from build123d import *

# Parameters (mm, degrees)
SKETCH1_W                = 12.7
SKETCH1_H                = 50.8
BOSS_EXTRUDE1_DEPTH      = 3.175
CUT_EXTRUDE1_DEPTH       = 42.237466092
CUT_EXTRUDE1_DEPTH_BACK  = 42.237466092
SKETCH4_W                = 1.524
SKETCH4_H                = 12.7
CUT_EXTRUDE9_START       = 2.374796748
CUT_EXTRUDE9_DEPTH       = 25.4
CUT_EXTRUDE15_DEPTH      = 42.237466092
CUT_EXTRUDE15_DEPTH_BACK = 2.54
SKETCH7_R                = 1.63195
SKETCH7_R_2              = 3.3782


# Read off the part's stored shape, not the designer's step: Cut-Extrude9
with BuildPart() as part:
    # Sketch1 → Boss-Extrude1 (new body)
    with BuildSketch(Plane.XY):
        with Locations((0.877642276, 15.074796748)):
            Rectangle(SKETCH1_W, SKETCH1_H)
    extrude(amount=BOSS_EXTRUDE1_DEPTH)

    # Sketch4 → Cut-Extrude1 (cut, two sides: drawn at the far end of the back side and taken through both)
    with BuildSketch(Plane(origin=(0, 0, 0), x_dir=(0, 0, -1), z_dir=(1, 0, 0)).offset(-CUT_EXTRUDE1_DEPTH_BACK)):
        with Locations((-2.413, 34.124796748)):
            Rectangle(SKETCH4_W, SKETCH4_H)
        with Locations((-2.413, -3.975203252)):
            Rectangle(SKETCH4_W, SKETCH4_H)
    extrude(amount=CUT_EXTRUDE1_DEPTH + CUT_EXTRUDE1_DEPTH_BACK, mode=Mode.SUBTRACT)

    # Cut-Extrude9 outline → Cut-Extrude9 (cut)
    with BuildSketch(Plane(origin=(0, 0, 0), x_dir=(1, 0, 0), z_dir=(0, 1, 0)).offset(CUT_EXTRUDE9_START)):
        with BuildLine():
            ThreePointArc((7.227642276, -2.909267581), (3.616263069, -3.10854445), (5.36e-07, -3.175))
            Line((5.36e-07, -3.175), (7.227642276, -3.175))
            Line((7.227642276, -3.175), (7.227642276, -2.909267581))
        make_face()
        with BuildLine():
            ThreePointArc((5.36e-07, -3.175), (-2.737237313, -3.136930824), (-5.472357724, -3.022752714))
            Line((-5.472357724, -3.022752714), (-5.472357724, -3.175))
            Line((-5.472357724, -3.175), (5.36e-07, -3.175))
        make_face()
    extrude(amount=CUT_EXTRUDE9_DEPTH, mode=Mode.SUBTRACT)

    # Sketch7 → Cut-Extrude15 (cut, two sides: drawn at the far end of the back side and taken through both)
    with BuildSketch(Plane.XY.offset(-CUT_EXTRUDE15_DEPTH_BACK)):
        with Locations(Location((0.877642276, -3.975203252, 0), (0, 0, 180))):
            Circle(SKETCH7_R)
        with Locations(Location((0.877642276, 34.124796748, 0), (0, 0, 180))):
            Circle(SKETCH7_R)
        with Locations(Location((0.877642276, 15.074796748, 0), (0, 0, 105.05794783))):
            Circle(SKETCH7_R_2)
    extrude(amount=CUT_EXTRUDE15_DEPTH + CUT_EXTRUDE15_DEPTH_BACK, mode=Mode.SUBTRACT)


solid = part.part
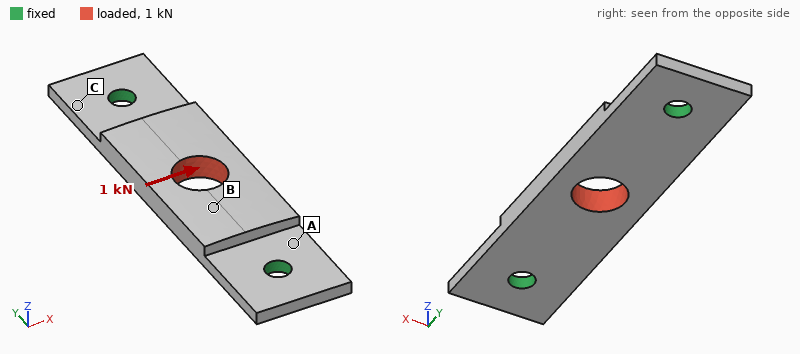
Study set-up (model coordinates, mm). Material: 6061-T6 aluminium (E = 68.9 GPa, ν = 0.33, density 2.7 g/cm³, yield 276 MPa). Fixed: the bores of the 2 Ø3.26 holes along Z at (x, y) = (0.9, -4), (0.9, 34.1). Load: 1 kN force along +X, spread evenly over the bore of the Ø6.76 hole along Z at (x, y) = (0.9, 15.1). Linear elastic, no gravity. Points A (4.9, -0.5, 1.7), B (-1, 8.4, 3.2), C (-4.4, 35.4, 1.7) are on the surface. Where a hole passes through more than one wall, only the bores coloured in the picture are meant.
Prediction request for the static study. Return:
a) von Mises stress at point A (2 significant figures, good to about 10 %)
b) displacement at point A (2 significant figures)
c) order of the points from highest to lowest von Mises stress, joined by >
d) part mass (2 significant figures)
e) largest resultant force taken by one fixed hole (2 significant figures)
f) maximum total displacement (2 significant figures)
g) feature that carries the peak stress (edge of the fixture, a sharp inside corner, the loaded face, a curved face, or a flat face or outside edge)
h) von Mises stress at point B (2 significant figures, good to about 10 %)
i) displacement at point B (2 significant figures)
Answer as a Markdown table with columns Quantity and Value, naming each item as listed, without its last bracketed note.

| Quantity | Value |
|---|---|
| von Mises stress at point A | 59 MPa |
| displacement at point A | 13 µm |
| order of the points from highest to lowest von Mises stress, joined by > | A > B > C |
| part mass | 3.8 g |
| largest resultant force taken by one fixed hole | 500 N |
| maximum total displacement | 47 µm |
| feature that carries the peak stress | edge of the fixture |
| von Mises stress at point B | 34 MPa |
| displacement at point B | 36 µm |
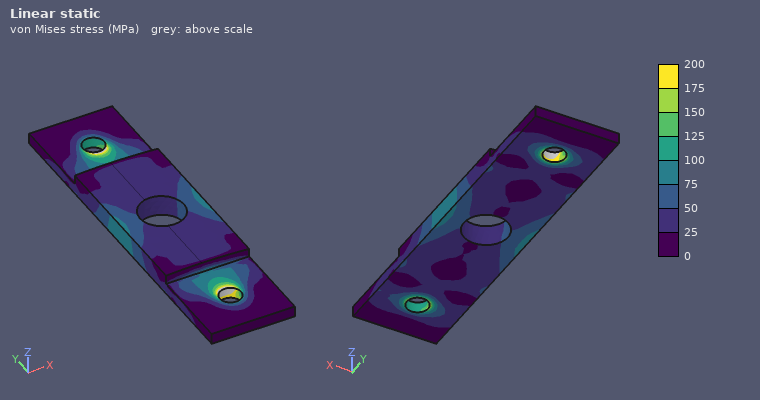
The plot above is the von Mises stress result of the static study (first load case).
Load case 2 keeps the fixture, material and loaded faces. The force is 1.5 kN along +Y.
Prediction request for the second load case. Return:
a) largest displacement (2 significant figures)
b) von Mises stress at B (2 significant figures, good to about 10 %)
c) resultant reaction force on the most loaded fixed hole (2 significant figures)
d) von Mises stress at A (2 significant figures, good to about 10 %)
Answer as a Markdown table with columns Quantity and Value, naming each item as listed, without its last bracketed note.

| Quantity | Value |
|---|---|
| largest displacement | 9.1 µm |
| von Mises stress at B | 13 MPa |
| resultant reaction force on the most loaded fixed hole | 750 N |
| von Mises stress at A | 36 MPa |
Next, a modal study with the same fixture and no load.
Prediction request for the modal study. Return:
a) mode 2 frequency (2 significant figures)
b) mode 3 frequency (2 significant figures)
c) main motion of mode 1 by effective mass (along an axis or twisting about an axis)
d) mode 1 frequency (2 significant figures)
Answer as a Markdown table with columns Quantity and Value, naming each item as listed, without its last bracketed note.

| Quantity | Value |
|---|---|
| mode 2 frequency | 11 kHz |
| mode 3 frequency | 20 kHz |
| main motion of mode 1 by effective mass | along Z |
| mode 1 frequency | 7700 Hz |
